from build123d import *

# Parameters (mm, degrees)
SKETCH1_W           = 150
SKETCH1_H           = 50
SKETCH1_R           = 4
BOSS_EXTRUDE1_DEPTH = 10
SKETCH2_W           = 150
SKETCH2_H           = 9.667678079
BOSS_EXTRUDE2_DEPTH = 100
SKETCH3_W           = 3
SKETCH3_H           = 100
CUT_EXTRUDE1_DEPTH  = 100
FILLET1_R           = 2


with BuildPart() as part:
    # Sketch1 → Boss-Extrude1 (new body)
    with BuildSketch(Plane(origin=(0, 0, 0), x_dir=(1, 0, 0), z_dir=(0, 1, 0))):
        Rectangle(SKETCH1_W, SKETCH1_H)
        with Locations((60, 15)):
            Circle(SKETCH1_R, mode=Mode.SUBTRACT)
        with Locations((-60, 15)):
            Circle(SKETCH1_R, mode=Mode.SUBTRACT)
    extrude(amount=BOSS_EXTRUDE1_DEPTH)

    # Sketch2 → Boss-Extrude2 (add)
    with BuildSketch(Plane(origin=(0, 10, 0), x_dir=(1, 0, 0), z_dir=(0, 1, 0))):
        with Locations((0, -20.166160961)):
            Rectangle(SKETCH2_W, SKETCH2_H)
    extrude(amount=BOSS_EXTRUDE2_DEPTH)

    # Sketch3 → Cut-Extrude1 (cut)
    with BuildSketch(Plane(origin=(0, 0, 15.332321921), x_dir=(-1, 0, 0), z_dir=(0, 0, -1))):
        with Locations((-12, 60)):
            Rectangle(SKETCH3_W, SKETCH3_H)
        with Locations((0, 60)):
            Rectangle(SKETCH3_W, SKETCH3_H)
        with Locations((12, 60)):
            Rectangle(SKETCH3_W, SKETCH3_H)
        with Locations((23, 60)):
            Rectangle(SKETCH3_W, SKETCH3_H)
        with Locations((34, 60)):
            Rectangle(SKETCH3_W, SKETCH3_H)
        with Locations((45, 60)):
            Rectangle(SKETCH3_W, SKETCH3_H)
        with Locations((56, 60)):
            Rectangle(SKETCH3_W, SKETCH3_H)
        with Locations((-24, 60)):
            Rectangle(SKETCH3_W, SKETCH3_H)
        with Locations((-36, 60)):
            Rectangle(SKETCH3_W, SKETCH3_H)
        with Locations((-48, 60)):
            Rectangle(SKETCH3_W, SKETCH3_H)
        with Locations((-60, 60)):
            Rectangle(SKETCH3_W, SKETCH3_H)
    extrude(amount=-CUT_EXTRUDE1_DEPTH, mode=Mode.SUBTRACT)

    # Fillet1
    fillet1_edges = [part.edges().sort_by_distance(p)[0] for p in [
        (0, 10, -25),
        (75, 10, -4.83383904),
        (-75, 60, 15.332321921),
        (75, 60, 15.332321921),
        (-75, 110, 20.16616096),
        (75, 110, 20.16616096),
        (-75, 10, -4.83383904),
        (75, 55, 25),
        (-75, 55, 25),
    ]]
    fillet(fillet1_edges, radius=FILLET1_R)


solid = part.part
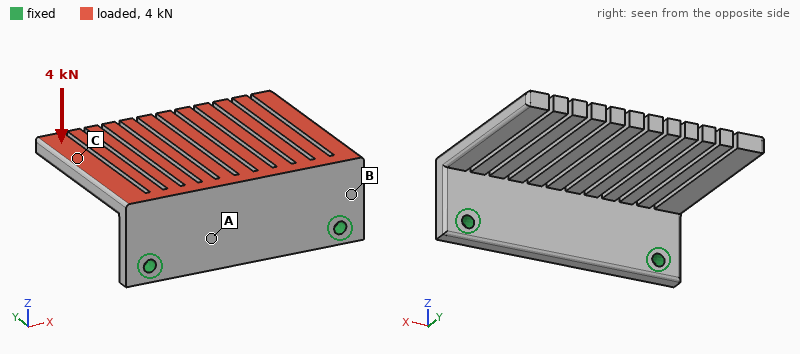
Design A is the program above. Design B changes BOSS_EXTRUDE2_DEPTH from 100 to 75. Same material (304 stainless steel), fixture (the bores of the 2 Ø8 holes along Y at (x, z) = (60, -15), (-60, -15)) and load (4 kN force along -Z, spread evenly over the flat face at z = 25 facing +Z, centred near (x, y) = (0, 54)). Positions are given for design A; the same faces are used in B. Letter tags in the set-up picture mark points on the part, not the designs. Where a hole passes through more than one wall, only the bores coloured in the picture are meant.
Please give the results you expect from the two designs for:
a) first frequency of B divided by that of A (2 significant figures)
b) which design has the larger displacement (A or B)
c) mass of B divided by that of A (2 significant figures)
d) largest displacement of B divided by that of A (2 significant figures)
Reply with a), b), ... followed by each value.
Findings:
a) 1.5
b) A
c) 0.85
d) 0.52
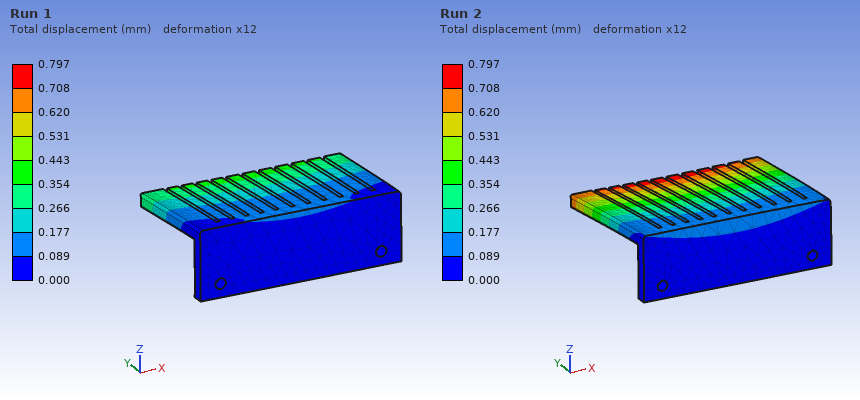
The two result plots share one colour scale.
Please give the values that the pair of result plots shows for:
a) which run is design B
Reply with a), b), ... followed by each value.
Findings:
a) Run 1
